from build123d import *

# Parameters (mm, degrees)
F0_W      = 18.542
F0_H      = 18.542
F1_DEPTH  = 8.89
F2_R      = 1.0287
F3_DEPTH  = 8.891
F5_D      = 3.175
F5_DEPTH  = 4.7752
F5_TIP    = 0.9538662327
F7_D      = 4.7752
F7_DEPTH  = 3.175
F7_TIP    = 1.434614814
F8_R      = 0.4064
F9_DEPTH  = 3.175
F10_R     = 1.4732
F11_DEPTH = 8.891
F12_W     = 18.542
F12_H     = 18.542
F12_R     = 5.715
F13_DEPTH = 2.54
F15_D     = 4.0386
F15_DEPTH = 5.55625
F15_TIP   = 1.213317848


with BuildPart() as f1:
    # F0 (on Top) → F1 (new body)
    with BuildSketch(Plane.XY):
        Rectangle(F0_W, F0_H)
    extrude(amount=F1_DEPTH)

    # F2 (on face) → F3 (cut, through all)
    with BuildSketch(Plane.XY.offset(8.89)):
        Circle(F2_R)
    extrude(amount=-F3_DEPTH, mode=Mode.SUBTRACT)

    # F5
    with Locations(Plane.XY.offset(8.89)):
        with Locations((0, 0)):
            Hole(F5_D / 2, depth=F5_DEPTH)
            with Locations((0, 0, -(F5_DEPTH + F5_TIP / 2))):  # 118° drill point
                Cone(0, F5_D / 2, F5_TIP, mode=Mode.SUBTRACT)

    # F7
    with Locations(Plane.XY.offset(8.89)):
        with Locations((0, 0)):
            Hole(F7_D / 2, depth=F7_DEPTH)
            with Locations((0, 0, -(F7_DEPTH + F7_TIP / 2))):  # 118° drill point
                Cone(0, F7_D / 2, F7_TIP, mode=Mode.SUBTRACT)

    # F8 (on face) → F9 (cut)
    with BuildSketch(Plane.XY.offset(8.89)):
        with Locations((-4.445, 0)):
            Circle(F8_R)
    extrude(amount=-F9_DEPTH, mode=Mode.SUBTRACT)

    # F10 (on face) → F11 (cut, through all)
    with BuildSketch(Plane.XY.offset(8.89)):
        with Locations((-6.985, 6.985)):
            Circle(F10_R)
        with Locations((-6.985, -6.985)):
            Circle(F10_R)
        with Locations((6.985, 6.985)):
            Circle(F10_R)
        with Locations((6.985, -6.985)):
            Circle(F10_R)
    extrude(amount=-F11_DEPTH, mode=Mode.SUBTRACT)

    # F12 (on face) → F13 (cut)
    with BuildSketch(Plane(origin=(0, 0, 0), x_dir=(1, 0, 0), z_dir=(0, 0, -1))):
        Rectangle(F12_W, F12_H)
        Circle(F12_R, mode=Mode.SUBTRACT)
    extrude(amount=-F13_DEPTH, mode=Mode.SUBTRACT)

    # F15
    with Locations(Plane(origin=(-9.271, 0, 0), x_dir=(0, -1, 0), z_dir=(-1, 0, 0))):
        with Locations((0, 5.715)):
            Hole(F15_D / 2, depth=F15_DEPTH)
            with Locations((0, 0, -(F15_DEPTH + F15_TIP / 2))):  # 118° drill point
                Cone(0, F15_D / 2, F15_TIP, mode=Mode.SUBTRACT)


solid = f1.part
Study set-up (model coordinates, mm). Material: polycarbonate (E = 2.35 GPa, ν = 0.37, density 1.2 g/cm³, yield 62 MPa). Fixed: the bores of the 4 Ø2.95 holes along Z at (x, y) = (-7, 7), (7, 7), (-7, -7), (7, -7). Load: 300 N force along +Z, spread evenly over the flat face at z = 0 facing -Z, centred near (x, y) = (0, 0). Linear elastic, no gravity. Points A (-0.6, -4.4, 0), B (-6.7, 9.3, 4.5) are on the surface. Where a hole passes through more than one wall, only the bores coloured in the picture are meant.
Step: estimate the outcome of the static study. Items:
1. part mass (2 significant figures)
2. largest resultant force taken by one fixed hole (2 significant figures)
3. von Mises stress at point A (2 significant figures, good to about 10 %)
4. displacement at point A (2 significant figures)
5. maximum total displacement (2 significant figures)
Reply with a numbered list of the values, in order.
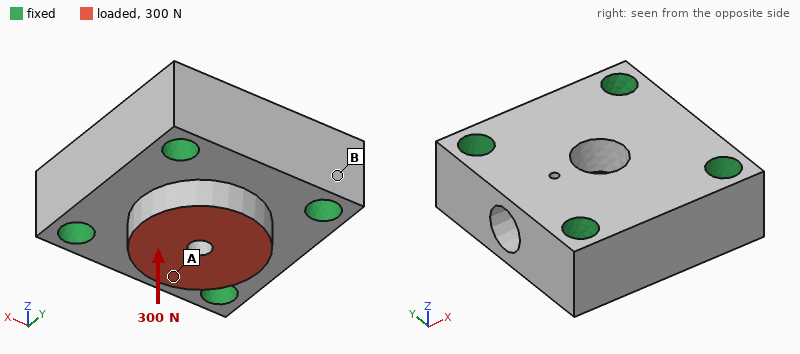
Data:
1. 2.5 g
2. 81 N
3. 2.4 MPa
4. 16 µm
5. 18 µm
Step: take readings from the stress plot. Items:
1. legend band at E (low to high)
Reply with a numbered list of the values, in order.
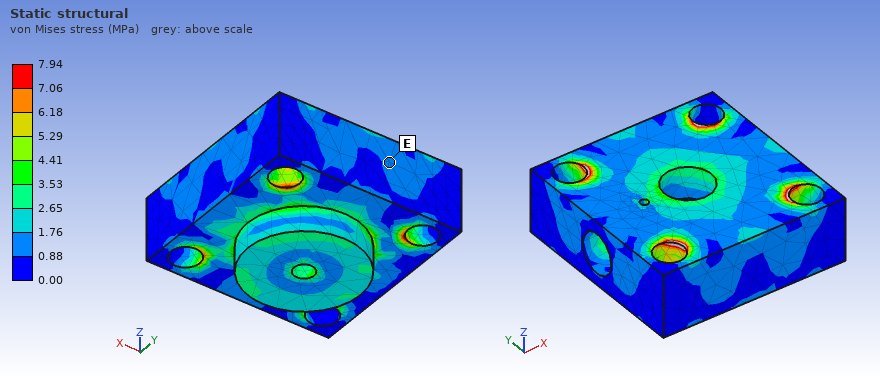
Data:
1. 0.88 to 1.76 MPa
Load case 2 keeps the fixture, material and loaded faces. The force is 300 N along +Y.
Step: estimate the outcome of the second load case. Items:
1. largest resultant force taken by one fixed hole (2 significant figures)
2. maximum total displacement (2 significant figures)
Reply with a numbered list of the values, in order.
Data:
1. 110 N
2. 36 µm
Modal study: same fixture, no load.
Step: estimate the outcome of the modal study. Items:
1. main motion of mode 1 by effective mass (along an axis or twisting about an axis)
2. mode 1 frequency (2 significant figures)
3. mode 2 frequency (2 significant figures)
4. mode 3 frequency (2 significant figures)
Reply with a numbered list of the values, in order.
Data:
1. along Z
2. 21 kHz
3. 25 kHz
4. 26 kHz
